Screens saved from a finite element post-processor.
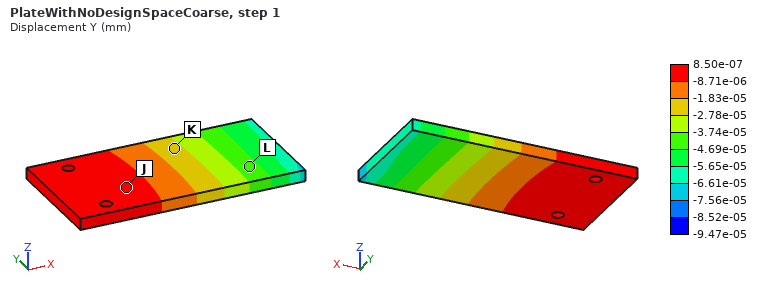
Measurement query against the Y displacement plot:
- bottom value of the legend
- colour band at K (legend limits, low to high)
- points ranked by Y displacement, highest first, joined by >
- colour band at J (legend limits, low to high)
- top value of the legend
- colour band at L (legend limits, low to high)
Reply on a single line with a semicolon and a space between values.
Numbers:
-9.47e-05 mm; -2.78e-05 to -1.83e-05 mm; J > K > L; -8.71e-06 to 8.50e-07 mm; 8.50e-07 mm; -4.69e-05 to -3.74e-05 mm
